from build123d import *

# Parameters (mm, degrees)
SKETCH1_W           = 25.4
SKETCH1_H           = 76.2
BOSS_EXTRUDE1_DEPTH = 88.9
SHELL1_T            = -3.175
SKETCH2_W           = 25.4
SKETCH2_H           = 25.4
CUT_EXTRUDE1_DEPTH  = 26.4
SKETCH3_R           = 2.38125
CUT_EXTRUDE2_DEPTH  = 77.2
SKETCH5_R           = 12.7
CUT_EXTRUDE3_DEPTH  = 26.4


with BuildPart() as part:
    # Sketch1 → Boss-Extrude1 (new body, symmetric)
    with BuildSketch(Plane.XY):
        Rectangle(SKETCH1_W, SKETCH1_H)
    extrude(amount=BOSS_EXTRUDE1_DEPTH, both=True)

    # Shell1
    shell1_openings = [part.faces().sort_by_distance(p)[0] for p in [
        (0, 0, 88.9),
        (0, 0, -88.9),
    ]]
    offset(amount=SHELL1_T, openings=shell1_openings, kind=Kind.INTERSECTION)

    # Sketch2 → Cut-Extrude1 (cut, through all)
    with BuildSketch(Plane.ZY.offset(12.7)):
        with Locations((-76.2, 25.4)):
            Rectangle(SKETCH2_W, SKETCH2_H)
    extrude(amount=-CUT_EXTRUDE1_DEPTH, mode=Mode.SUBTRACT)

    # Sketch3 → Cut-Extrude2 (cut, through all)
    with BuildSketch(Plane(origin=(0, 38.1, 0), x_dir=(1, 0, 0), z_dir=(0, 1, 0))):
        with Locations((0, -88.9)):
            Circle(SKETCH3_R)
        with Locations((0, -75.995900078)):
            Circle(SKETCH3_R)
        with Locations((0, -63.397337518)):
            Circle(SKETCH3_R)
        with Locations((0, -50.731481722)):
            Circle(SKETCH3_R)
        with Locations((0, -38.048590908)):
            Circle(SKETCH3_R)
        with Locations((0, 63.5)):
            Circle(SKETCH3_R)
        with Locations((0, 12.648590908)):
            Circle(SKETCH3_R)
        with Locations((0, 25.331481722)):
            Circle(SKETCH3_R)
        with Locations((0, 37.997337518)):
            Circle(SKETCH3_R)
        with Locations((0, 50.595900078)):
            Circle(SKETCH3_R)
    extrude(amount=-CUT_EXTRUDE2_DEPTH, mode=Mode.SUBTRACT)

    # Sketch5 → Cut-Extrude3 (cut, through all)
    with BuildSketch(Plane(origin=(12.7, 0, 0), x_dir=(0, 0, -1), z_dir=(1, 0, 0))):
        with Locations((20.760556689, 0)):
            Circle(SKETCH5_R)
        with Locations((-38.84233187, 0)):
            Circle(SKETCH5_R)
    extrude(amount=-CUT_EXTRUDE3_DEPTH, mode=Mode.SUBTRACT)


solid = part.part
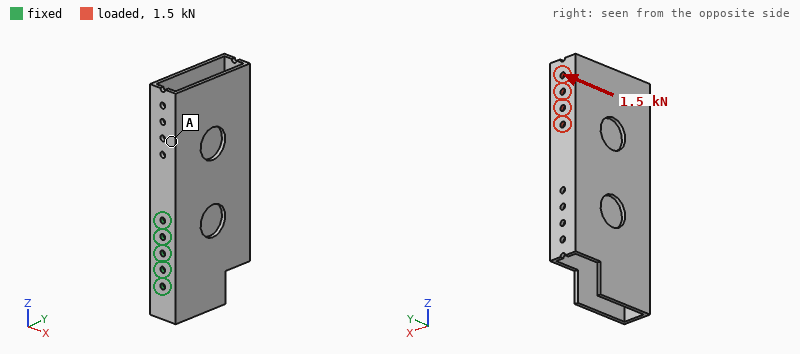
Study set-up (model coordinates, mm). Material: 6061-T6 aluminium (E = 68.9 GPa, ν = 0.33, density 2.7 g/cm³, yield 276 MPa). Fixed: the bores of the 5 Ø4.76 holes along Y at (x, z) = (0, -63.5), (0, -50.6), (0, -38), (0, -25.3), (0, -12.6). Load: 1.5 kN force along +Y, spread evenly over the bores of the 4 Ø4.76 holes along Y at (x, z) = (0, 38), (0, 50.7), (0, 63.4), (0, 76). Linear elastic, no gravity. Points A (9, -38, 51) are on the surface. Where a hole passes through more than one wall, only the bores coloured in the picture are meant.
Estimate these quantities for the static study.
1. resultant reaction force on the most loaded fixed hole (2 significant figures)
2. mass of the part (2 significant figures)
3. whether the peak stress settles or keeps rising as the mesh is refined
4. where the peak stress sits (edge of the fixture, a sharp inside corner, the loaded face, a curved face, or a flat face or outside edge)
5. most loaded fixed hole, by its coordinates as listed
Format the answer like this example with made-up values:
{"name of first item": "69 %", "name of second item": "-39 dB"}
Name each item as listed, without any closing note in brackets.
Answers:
{"resultant reaction force on the most loaded fixed hole": "2.8 kN", "mass of the part": "250 g", "whether the peak stress settles or keeps rising as the mesh is refined": "keeps rising", "where the peak stress sits": "edge of the fixture", "most loaded fixed hole, by its coordinates as listed": "(0, -12.6)"}
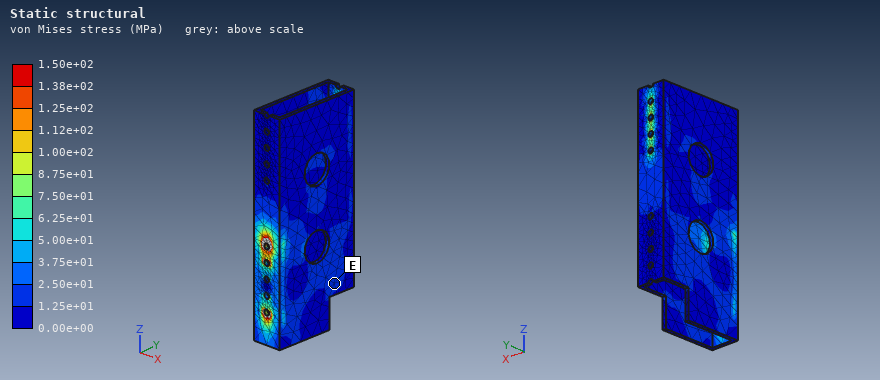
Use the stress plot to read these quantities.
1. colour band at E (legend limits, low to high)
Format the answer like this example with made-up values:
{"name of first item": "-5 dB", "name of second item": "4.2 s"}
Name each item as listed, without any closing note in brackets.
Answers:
{"colour band at E": "1.25e+01 to 2.50e+01 MPa"}
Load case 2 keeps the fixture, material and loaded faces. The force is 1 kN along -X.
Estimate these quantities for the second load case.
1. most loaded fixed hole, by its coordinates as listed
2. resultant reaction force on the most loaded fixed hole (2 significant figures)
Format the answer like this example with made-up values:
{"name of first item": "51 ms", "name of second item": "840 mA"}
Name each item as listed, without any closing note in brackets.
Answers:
{"most loaded fixed hole, by its coordinates as listed": "(0, -12.6)", "resultant reaction force on the most loaded fixed hole": "2.7 kN"}
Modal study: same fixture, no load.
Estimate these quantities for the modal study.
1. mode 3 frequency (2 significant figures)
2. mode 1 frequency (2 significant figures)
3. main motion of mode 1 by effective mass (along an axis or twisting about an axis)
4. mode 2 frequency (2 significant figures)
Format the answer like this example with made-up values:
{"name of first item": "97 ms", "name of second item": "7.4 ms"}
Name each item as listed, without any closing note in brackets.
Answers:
{"mode 3 frequency": "980 Hz", "mode 1 frequency": "410 Hz", "main motion of mode 1 by effective mass": "along X", "mode 2 frequency": "910 Hz"}
